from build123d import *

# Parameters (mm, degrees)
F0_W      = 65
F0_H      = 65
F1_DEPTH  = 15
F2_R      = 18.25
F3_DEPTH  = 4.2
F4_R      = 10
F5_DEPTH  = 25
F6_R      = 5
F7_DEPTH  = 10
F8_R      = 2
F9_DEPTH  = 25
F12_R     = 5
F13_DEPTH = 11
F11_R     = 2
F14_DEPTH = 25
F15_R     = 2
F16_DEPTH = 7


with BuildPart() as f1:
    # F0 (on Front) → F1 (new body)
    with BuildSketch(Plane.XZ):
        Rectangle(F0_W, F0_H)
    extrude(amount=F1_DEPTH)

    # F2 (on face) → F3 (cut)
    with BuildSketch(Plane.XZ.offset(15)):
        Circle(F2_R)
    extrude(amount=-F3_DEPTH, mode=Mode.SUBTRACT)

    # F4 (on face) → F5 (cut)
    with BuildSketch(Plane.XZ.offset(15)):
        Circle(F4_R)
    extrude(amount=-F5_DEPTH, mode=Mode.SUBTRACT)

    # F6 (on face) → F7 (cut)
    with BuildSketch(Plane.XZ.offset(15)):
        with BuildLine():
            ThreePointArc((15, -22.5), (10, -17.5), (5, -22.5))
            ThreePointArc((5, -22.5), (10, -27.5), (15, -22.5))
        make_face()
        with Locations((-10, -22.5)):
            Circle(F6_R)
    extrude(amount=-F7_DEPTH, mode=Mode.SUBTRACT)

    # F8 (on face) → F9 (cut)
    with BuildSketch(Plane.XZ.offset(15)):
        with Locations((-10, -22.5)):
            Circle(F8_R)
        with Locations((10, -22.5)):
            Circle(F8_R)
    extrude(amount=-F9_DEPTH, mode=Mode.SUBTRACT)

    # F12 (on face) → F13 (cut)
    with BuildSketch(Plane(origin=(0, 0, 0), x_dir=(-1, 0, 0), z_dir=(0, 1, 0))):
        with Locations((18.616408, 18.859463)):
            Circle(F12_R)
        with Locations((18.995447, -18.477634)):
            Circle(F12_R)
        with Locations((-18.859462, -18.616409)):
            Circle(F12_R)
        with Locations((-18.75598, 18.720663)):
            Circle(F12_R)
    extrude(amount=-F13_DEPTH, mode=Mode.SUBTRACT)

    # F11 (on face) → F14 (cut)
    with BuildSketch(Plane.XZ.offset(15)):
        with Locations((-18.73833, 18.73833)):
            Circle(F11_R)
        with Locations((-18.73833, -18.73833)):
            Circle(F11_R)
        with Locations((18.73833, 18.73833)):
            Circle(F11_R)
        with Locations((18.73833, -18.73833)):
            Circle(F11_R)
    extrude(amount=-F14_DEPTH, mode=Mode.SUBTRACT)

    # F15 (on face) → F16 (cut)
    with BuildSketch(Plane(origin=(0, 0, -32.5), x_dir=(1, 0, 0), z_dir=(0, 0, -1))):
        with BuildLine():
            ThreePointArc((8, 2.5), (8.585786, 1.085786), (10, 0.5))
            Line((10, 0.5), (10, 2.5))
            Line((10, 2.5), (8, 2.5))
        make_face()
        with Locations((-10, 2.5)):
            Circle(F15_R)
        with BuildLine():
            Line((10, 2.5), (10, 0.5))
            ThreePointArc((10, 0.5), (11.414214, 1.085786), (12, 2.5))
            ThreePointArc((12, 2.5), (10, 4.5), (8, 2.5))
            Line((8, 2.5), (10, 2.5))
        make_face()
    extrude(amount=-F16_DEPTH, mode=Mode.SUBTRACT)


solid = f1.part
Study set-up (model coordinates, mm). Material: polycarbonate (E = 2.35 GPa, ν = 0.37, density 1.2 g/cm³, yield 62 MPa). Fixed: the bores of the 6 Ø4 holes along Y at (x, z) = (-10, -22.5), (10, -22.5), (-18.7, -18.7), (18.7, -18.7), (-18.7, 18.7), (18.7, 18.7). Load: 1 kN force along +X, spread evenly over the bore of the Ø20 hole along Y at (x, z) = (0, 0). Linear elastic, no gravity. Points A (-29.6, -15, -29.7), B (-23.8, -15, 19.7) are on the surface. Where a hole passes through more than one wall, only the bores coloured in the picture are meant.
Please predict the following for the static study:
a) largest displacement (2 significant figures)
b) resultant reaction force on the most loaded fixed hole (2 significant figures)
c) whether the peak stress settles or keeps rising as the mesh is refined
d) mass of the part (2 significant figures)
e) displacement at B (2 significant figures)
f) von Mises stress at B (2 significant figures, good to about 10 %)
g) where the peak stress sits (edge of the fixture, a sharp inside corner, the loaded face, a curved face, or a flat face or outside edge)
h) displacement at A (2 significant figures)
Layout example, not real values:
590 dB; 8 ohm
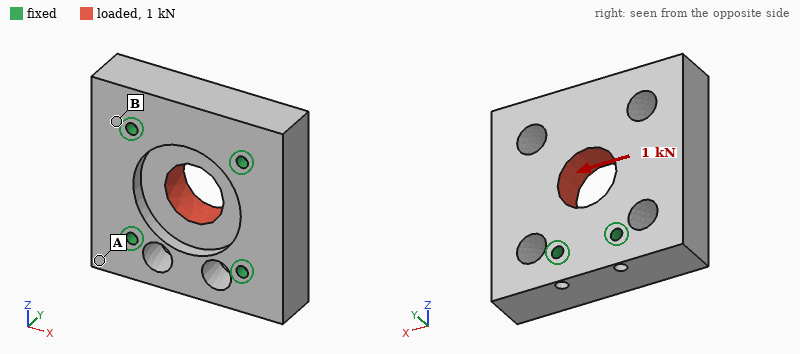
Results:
37 µm; 250 N; keeps rising; 60 g; 7.2 µm; 2.0 MPa; edge of the fixture; 10 µm
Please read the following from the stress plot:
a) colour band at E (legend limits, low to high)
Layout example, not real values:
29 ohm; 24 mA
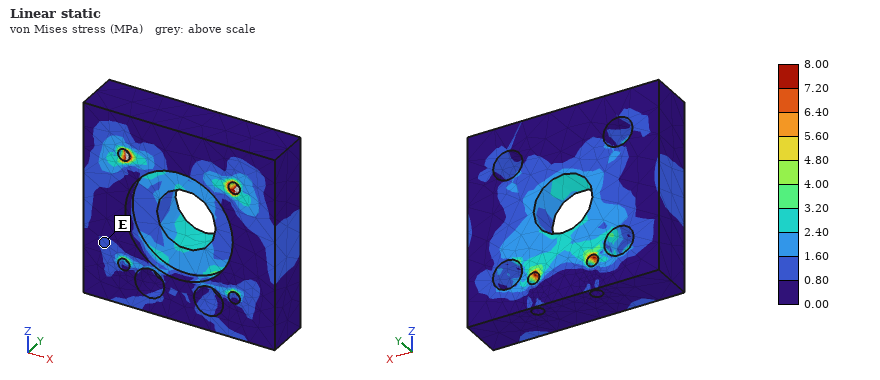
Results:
0.80 to 1.60 MPa
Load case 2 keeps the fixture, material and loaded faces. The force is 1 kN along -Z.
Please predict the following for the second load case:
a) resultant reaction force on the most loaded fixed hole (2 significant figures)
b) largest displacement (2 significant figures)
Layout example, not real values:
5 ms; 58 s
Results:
200 N; 39 µm
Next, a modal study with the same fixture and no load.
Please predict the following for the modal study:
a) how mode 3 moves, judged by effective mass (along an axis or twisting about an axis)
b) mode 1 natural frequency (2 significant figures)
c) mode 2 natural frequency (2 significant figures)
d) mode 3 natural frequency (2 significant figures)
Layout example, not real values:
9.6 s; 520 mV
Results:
along Y; 3700 Hz; 3800 Hz; 4200 Hz
